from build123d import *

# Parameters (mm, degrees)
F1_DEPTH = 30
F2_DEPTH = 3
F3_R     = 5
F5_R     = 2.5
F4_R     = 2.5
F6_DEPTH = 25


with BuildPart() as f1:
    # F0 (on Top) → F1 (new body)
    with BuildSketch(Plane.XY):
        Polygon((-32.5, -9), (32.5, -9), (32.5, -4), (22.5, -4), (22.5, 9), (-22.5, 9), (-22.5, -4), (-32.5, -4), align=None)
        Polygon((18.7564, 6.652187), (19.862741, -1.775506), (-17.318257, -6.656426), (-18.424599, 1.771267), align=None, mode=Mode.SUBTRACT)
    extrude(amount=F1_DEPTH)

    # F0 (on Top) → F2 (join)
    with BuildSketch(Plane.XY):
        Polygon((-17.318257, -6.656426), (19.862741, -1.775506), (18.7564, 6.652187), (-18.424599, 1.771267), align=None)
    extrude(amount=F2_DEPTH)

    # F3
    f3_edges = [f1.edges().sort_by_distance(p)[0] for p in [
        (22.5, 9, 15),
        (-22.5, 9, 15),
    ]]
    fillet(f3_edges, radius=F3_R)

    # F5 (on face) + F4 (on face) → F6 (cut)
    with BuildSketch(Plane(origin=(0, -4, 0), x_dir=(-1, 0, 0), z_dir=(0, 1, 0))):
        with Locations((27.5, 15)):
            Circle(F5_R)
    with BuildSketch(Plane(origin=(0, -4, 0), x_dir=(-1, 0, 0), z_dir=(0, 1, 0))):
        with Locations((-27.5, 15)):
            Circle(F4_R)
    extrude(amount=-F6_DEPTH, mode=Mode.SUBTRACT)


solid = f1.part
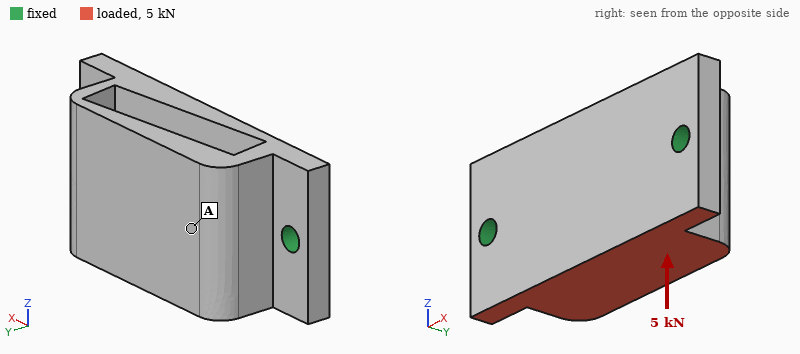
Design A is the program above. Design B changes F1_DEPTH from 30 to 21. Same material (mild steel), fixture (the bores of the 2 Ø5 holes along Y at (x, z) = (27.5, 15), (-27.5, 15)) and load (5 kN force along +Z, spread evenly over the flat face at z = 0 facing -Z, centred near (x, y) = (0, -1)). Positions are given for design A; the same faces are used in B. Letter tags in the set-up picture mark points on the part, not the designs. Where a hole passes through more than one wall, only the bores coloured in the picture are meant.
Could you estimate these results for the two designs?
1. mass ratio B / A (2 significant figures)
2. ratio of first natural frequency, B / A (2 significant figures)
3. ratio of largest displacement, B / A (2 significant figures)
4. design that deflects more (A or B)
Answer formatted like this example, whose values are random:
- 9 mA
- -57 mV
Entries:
- 0.71
- 1.1
- 1.3
- B
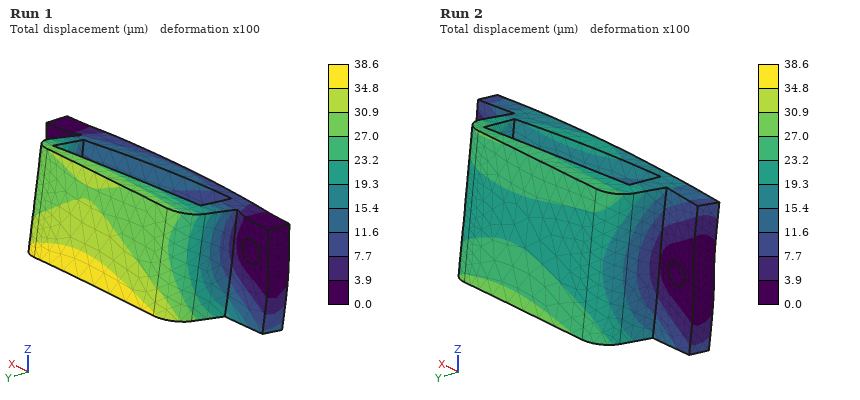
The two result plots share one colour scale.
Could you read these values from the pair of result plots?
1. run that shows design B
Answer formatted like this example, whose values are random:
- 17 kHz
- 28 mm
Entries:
- Run 1
